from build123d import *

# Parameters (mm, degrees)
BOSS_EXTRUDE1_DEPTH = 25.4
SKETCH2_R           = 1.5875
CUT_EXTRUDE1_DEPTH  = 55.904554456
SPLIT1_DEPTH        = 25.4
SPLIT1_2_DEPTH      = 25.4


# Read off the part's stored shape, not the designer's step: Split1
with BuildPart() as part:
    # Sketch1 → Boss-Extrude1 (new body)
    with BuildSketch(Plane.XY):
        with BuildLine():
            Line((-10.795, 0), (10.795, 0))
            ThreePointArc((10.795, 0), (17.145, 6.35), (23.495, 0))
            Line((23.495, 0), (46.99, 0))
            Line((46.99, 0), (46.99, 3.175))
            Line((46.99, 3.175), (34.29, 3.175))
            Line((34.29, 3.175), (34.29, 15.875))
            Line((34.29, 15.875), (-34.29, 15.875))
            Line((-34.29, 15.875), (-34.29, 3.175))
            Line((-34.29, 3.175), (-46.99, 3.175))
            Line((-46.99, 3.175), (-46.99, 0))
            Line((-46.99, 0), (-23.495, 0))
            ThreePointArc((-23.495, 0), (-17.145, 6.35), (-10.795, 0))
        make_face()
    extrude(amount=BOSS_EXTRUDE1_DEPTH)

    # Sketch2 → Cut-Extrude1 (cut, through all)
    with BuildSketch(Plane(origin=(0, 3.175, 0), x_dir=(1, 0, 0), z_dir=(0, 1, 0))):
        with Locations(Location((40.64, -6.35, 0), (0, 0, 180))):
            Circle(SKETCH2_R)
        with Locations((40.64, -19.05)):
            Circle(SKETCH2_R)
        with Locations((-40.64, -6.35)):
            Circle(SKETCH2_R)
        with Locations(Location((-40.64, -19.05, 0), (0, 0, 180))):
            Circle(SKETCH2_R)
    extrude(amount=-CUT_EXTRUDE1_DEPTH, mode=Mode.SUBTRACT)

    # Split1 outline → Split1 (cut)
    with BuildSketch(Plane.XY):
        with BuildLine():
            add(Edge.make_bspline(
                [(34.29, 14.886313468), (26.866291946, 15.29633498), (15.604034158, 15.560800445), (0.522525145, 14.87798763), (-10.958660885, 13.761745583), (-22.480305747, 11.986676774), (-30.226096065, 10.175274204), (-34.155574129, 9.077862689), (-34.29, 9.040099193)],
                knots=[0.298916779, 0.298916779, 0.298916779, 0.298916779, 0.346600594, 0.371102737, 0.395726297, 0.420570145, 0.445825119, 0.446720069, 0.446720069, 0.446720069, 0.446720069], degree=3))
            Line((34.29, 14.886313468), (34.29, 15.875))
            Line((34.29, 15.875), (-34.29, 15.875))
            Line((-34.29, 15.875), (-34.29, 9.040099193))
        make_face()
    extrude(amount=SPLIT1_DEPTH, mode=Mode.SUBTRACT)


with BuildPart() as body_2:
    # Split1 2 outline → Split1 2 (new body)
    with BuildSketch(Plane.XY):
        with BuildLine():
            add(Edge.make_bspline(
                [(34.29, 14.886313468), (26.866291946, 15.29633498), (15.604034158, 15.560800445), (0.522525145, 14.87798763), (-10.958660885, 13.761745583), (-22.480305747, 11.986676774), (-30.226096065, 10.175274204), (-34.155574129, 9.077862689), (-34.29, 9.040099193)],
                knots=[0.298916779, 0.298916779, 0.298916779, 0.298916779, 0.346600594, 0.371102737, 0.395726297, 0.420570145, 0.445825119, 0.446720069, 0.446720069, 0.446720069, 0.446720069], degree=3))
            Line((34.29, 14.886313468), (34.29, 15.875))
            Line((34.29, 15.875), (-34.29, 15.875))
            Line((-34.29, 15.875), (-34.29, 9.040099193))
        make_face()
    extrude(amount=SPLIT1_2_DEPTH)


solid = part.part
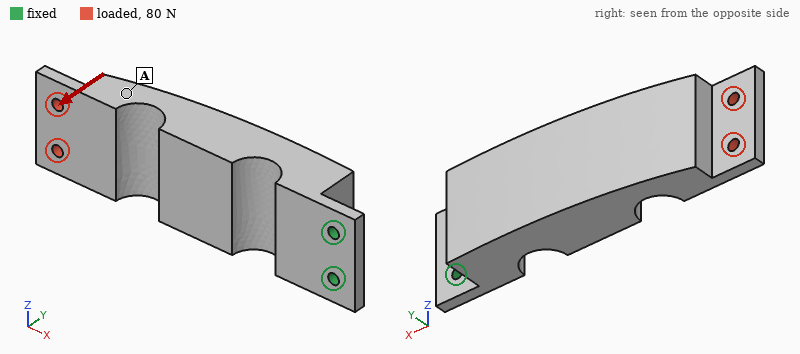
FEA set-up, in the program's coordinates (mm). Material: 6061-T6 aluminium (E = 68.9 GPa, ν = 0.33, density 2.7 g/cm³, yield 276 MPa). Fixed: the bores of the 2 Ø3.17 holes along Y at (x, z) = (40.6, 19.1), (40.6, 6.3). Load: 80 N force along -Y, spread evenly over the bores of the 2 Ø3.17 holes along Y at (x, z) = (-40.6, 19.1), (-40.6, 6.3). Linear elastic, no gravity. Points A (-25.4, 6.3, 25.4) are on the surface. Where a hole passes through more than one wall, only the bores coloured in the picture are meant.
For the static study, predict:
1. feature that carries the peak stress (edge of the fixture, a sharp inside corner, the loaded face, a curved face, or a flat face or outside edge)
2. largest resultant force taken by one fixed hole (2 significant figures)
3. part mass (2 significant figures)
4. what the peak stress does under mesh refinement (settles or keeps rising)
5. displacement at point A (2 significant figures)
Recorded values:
edge of the fixture
41 N
62 g
keeps rising
0.64 mm
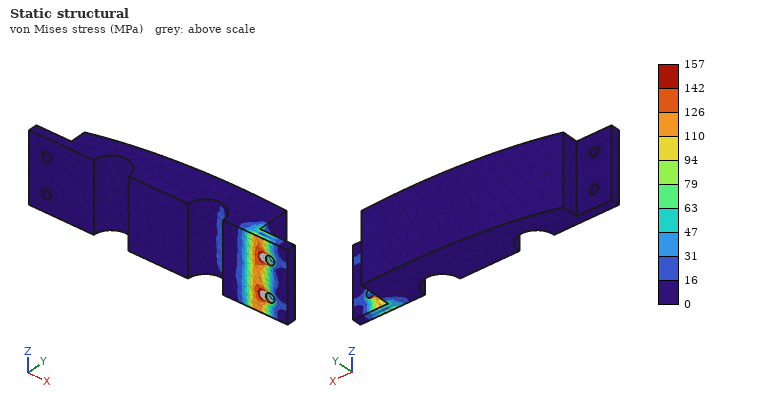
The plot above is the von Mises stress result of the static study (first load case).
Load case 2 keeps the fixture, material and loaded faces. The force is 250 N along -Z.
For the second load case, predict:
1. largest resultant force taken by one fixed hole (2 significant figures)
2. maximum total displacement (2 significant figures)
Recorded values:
1.4 kN
0.15 mm
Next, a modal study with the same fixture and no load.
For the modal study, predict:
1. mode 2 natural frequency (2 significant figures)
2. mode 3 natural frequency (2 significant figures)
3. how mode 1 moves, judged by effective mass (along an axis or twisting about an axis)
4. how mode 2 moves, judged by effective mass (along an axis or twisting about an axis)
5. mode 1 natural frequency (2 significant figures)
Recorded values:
1800 Hz
3900 Hz
along Y
along Z
380 Hz
